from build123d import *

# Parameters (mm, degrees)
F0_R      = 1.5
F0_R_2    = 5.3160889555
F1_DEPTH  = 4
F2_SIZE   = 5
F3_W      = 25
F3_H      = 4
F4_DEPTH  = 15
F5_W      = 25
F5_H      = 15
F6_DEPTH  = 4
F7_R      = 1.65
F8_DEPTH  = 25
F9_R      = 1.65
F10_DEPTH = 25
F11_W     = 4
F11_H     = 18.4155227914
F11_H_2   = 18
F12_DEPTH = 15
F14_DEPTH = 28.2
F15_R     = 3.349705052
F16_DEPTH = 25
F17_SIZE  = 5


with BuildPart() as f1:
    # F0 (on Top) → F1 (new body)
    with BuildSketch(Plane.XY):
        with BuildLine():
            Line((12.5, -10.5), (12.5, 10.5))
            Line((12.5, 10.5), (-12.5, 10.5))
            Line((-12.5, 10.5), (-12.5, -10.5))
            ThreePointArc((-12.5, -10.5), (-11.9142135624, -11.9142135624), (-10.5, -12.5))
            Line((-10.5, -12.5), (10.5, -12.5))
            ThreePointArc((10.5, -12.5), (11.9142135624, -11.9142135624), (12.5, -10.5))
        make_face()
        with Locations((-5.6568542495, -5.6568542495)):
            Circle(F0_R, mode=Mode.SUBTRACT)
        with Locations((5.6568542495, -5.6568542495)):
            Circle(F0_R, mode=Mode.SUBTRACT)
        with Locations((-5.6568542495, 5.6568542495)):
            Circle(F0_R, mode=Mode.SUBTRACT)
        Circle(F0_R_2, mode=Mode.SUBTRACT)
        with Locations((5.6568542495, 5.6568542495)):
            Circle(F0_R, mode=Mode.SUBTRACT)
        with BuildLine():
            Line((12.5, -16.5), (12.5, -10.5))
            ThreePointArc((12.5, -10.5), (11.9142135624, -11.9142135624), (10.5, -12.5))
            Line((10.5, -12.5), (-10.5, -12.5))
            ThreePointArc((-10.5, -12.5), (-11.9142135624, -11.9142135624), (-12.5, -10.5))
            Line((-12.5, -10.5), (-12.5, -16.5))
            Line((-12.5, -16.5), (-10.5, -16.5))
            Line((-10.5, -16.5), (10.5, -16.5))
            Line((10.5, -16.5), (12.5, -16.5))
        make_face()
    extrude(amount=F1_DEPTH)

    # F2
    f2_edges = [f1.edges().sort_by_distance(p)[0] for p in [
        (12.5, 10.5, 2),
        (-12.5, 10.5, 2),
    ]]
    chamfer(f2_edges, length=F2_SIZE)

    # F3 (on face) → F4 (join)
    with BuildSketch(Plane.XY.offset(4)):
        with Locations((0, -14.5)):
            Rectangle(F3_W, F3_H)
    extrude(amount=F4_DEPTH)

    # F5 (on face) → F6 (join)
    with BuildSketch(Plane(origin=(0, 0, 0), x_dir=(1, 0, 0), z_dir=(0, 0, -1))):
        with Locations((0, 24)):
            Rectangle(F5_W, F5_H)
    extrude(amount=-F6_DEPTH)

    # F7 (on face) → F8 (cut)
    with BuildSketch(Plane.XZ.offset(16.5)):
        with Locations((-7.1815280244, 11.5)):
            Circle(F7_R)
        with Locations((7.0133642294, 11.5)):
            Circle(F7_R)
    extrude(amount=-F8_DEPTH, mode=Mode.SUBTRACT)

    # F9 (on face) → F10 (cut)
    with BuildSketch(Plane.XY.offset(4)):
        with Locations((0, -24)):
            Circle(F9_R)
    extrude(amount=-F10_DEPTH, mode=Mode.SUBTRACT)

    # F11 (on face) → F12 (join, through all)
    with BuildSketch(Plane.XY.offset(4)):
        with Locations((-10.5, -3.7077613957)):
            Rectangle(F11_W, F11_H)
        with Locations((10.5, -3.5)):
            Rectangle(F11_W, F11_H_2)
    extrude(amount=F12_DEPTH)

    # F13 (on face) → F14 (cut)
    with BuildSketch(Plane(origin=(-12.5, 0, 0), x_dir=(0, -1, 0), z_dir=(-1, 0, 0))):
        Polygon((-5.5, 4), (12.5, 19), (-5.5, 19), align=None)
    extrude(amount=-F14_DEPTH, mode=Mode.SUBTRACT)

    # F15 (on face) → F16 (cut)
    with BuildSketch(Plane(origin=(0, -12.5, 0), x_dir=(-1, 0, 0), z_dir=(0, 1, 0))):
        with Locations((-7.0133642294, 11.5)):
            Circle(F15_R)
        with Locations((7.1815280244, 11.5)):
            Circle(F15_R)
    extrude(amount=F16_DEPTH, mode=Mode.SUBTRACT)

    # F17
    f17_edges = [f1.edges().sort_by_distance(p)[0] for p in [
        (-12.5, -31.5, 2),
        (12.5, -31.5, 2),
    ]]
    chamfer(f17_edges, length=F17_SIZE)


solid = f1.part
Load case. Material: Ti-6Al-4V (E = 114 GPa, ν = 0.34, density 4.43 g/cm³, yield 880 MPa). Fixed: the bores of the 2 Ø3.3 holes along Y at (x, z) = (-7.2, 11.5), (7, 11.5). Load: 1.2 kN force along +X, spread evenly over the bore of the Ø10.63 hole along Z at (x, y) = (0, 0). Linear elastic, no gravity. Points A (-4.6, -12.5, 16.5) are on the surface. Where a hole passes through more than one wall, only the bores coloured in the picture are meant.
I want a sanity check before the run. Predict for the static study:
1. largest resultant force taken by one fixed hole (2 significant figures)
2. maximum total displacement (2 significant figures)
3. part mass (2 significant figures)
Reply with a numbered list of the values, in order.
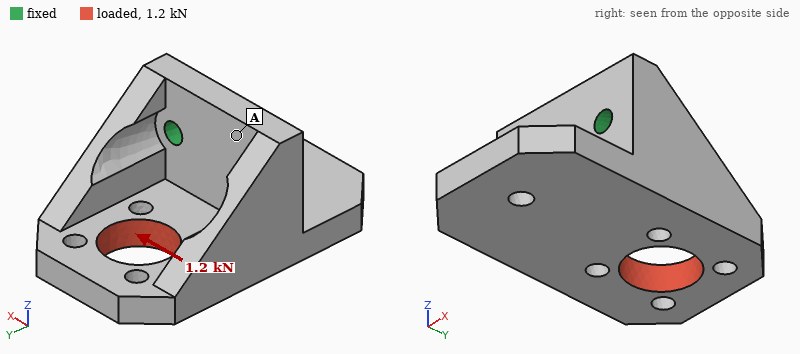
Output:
1. 1.2 kN
2. 47 µm
3. 26 g
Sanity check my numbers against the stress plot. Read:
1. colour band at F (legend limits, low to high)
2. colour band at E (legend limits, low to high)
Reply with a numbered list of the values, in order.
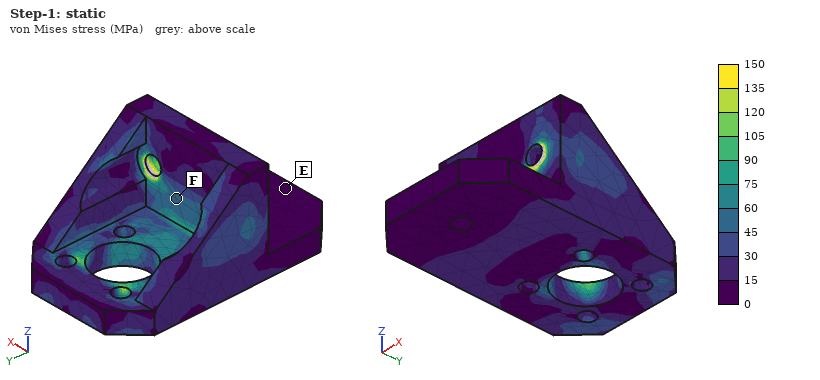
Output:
1. 45 to 60 MPa
2. 0 to 15 MPa
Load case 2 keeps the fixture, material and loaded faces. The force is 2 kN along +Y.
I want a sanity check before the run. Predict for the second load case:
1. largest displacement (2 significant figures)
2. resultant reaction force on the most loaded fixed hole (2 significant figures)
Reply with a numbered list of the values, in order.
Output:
1. 77 µm
2. 1.0 kN
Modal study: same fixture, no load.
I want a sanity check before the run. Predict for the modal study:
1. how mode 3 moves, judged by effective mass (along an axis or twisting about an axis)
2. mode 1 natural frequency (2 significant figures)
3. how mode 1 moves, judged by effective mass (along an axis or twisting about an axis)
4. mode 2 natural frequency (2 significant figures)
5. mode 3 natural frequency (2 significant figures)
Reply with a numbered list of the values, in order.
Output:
1. along Z
2. 6200 Hz
3. along Y
4. 8800 Hz
5. 13 kHz
